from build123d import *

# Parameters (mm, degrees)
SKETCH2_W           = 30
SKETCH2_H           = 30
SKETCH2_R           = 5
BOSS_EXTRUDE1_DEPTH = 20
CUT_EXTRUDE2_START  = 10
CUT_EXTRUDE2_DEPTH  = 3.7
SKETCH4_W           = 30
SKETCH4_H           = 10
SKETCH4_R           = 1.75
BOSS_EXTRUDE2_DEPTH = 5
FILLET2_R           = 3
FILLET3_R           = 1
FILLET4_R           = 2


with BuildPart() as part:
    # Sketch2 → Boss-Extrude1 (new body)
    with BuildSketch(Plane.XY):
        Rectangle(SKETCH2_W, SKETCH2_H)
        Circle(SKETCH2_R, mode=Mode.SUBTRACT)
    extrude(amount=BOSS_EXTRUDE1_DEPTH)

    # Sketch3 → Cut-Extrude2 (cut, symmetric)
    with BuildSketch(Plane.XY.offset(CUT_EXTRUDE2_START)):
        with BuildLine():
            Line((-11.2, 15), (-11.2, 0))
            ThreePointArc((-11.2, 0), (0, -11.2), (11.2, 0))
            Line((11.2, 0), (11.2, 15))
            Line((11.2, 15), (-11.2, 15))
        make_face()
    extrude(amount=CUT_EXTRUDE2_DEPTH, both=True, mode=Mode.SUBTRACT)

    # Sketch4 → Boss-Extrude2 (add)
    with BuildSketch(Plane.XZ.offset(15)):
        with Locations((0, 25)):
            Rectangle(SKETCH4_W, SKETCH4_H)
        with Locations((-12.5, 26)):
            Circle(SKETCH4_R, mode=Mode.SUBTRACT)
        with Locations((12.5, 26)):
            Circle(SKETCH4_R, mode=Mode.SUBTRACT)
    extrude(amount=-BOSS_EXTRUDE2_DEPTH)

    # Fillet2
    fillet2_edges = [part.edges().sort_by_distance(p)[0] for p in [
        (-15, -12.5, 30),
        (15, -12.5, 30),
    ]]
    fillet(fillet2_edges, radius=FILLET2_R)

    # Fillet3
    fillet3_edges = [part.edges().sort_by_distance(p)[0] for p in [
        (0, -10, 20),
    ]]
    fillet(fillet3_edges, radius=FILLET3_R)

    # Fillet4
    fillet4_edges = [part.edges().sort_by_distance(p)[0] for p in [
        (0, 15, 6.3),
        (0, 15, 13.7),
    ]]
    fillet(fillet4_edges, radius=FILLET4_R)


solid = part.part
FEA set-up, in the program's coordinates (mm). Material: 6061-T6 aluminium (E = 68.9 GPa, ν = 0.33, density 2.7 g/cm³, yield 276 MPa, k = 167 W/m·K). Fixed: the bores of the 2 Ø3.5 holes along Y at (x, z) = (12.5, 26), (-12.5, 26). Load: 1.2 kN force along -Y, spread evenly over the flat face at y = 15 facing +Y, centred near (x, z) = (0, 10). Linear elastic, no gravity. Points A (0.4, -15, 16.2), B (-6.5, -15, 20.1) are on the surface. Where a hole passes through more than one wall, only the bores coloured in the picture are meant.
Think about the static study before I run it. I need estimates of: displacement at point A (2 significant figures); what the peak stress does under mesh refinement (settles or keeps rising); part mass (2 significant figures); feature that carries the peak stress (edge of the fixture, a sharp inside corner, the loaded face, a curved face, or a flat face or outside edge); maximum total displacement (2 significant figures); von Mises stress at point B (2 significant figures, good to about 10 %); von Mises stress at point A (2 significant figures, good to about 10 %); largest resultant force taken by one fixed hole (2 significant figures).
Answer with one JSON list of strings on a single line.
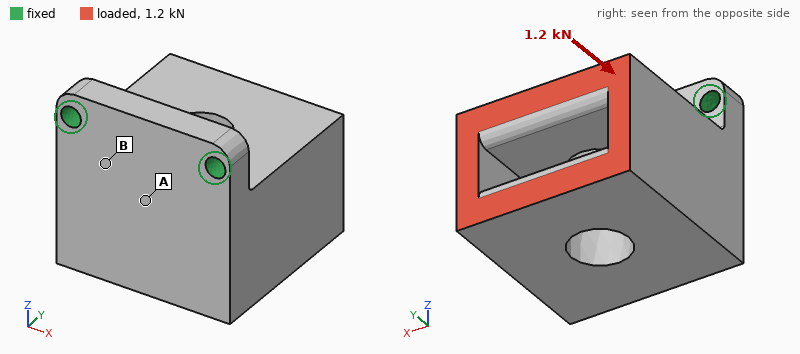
["0.049 mm", "keeps rising", "39 g", "edge of the fixture", "0.24 mm", "69 MPa", "29 MPa", "600 N"]
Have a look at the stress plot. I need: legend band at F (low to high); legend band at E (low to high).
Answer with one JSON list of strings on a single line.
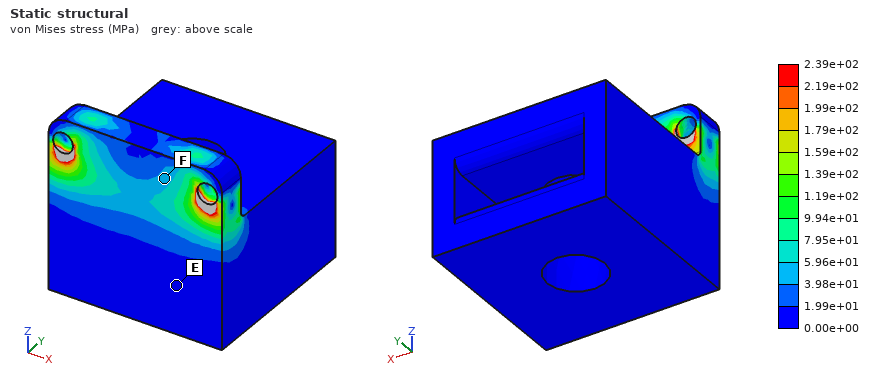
["3.98e+01 to 5.96e+01 MPa", "0.00e+00 to 1.99e+01 MPa"]
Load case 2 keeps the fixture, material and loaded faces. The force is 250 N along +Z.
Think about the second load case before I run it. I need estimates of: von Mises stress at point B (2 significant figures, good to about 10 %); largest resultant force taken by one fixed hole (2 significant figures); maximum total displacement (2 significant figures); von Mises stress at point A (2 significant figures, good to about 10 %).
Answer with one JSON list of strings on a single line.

["38 MPa", "130 N", "0.11 mm", "17 MPa"]
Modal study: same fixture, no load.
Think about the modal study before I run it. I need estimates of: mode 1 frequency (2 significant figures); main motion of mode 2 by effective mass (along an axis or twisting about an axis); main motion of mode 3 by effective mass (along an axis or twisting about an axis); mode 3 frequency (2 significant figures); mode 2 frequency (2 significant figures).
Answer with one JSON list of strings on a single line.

["2000 Hz", "along X", "along X", "12 kHz", "5900 Hz"]
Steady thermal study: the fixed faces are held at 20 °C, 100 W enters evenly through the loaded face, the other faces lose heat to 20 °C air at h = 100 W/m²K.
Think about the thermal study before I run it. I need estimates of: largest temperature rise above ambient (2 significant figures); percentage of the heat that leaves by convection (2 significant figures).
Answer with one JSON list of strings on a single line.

["75 K", "27 %"]
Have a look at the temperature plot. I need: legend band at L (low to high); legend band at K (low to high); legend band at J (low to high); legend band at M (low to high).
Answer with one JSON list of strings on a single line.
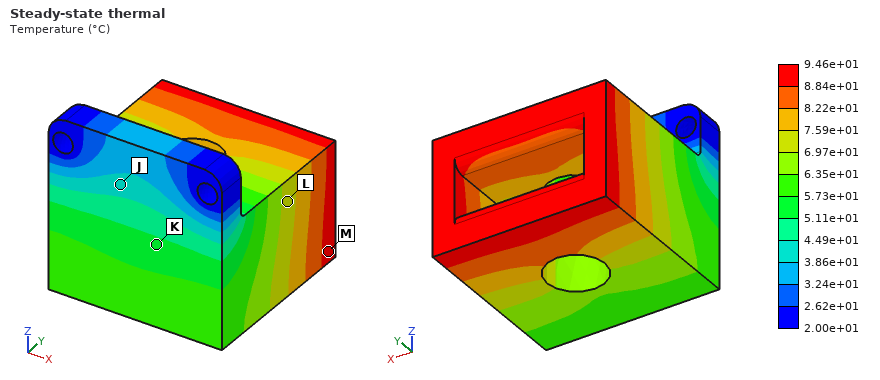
["6.97e+01 to 7.59e+01 °C", "5.11e+01 to 5.73e+01 °C", "3.86e+01 to 4.49e+01 °C", "8.84e+01 to 9.46e+01 °C"]
